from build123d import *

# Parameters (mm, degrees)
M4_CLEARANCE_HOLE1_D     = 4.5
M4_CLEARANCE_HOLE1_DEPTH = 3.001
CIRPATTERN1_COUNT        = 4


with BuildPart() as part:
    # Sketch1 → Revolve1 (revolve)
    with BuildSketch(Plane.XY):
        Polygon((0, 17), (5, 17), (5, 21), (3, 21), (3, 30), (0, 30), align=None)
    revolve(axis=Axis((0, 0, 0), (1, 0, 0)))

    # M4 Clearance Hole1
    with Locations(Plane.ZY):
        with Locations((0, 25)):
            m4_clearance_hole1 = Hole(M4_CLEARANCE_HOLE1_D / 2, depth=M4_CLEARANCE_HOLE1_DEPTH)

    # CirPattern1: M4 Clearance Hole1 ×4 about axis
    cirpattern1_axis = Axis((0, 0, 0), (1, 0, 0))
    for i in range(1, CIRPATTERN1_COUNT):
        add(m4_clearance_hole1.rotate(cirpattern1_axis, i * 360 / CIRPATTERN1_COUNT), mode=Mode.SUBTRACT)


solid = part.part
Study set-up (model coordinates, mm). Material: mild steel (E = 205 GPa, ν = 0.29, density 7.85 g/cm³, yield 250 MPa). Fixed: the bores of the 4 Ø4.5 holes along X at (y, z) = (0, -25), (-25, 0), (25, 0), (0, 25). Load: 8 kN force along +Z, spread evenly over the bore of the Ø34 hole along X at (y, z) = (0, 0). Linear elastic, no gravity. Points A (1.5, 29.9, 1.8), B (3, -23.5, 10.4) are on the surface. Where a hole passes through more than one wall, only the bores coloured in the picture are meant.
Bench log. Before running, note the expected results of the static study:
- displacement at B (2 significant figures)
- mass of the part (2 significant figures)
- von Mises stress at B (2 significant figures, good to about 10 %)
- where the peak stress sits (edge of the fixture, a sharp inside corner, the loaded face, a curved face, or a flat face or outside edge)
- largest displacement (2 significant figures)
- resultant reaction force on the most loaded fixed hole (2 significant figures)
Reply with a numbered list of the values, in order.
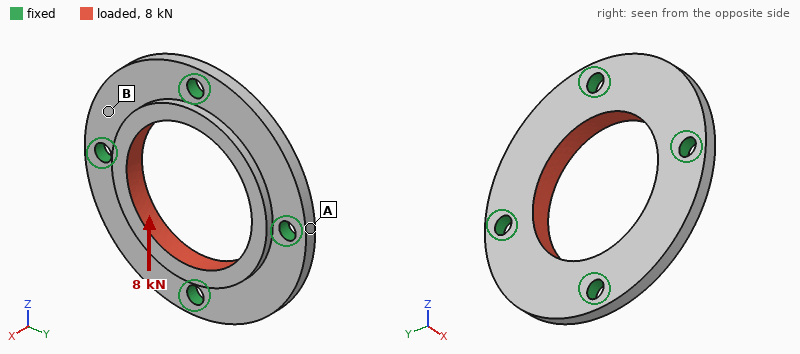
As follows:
1. 2.8 µm
2. 51 g
3. 28 MPa
4. edge of the fixture
5. 5.8 µm
6. 2.3 kN
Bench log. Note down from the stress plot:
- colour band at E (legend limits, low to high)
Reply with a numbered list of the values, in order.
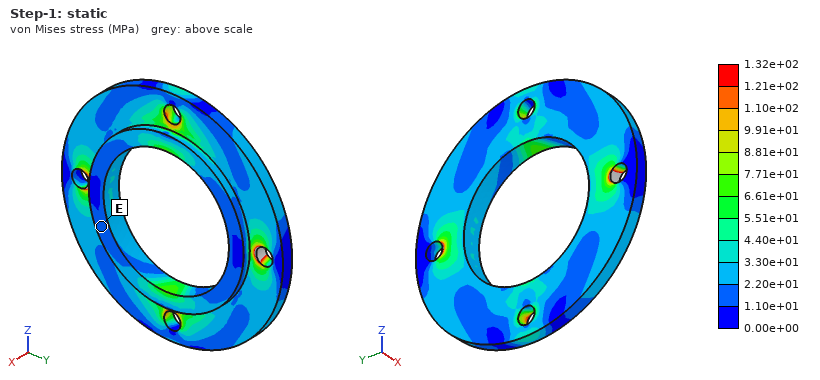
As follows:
1. 1.10e+01 to 2.20e+01 MPa
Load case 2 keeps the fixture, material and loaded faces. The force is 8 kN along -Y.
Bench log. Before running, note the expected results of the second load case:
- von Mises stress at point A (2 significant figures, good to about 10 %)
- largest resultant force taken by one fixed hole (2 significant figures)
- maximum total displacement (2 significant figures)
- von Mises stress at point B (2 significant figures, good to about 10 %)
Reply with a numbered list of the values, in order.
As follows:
1. 35 MPa
2. 2.3 kN
3. 5.8 µm
4. 26 MPa
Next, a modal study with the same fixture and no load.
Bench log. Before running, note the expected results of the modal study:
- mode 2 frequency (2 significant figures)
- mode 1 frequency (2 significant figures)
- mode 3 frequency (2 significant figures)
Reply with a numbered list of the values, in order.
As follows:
1. 12 kHz
2. 11 kHz
3. 12 kHz
